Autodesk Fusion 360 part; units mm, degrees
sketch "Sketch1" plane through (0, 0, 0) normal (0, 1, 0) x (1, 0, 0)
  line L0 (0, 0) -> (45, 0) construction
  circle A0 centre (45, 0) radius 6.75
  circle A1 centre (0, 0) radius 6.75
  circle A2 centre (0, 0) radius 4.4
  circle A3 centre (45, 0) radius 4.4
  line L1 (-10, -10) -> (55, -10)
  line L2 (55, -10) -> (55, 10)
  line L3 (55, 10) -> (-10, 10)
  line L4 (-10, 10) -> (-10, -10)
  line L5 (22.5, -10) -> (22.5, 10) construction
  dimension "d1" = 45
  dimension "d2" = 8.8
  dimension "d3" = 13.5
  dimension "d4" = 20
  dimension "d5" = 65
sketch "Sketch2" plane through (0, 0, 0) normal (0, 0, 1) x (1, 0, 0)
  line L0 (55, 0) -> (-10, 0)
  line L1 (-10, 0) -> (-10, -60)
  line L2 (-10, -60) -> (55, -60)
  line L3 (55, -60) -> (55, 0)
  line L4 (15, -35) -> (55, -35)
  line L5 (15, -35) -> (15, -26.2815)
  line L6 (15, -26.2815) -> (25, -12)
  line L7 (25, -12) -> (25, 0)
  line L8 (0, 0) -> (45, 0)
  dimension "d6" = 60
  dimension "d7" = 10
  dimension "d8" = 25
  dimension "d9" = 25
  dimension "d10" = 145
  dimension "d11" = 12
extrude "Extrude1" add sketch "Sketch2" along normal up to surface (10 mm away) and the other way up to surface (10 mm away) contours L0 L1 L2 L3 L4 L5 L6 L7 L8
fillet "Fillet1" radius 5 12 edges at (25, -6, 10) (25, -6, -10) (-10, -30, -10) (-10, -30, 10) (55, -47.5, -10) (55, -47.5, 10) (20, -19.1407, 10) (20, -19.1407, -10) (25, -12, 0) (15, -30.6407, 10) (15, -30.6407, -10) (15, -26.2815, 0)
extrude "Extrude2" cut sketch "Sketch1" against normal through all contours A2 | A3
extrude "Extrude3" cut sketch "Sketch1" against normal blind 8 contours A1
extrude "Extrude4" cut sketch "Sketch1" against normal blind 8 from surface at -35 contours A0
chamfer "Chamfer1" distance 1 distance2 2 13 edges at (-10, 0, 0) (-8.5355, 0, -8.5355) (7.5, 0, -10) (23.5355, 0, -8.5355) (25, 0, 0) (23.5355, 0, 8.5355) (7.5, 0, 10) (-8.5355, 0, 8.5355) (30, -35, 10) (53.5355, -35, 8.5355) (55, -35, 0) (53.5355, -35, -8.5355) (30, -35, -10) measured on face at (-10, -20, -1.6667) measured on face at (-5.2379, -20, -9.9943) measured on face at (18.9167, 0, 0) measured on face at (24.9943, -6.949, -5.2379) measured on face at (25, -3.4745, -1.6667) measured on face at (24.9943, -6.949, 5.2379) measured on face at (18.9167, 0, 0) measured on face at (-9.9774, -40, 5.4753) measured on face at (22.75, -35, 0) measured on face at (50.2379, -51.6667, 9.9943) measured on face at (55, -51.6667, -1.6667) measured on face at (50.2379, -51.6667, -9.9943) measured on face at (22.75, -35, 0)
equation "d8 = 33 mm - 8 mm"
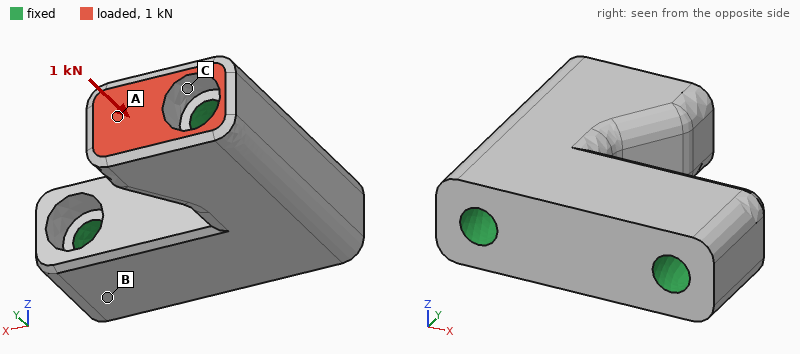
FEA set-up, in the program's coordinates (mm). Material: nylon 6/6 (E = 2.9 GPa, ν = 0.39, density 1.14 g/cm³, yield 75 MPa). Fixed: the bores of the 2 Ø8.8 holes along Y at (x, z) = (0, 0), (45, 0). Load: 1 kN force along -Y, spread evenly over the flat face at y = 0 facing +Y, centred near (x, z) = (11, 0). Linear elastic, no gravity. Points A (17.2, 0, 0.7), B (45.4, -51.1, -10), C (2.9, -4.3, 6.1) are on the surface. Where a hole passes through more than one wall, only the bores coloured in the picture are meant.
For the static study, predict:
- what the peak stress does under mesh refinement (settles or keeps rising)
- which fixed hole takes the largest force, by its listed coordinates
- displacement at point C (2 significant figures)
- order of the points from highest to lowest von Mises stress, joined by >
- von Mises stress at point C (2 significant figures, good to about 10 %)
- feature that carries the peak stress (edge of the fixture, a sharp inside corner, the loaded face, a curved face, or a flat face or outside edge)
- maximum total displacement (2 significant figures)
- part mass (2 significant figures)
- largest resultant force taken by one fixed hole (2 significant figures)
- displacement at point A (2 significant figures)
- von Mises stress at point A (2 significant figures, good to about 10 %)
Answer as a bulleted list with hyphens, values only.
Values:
- keeps rising
- (0, 0)
- 17 µm
- C > A > B
- 3.7 MPa
- edge of the fixture
- 51 µm
- 52 g
- 980 N
- 46 µm
- 1.8 MPa
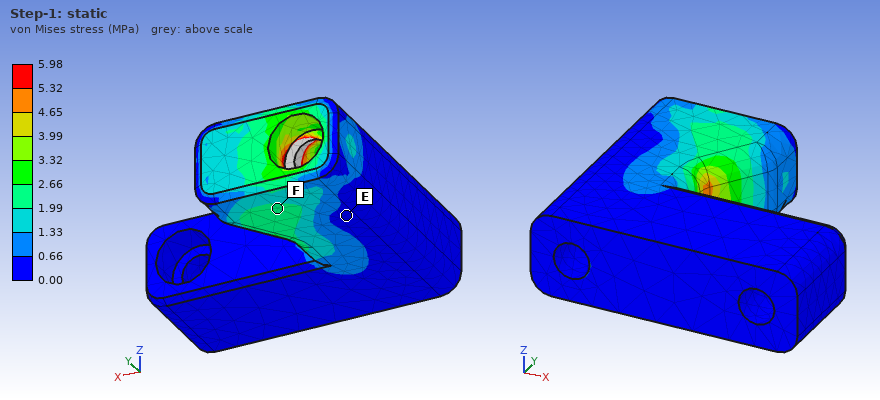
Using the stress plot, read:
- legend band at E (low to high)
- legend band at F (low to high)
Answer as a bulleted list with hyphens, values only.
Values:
- 0.00 to 0.66 MPa
- 1.99 to 2.66 MPa
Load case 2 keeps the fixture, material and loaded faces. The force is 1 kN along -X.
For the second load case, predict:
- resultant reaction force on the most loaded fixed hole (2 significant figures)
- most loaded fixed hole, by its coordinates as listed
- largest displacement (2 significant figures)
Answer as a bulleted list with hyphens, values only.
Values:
- 1000 N
- (0, 0)
- 0.11 mm
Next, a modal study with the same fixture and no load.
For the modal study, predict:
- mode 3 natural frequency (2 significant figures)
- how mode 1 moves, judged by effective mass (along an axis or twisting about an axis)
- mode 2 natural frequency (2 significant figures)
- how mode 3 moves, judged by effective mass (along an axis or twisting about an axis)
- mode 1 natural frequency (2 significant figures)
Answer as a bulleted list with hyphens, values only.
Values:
- 8400 Hz
- along Z
- 7800 Hz
- along Z
- 5800 Hz
